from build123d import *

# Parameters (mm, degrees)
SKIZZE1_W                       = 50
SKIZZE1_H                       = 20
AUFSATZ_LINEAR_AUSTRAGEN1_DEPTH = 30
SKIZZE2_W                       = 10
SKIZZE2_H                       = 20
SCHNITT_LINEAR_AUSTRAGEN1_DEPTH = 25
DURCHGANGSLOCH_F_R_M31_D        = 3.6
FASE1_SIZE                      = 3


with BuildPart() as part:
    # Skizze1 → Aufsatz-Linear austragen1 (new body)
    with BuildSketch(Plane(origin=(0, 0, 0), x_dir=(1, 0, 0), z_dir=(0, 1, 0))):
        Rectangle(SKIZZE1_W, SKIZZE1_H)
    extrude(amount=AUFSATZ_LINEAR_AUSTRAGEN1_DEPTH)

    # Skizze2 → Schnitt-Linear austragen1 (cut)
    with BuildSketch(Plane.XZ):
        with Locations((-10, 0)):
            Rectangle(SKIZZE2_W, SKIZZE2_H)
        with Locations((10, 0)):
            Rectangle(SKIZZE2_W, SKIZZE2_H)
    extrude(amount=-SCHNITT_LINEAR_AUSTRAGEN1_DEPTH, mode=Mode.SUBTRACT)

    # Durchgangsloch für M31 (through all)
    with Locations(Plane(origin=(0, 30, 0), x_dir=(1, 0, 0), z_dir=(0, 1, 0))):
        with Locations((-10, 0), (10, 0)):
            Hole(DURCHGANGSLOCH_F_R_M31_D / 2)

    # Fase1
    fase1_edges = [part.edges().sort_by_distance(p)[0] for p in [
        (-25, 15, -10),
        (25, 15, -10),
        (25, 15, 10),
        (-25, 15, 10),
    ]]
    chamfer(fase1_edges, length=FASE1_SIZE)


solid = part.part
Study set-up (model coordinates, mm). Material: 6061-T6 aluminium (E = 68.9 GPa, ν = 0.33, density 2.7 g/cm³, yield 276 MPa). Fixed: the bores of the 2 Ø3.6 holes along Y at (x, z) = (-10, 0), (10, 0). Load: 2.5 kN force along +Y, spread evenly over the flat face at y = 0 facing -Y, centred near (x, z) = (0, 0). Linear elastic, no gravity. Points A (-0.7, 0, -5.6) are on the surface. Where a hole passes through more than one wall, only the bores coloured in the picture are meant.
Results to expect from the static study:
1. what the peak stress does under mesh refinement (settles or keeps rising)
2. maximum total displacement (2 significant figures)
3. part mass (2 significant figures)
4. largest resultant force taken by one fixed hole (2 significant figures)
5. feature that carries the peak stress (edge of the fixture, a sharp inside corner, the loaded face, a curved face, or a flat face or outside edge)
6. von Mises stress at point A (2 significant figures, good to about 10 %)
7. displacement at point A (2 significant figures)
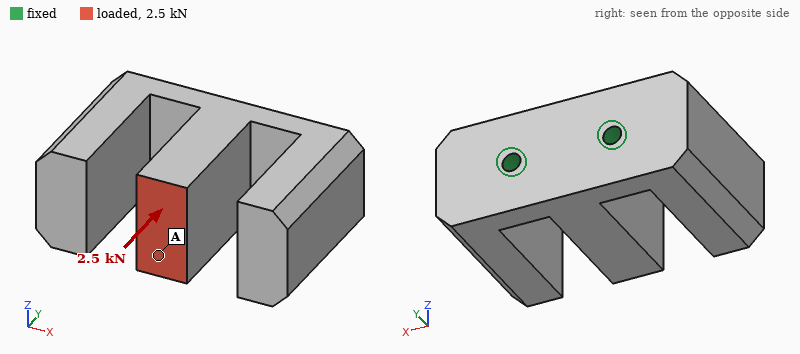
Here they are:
keeps rising
14 µm
52 g
1.3 kN
edge of the fixture
12 MPa
13 µm
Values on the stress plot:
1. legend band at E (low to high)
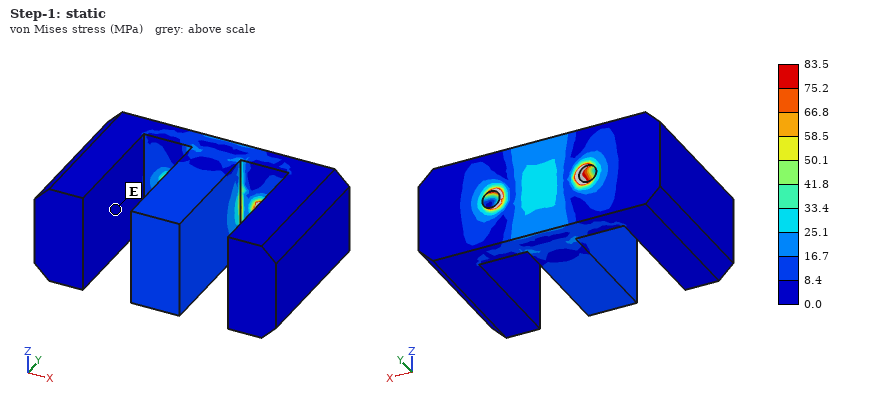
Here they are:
0.0 to 8.4 MPa
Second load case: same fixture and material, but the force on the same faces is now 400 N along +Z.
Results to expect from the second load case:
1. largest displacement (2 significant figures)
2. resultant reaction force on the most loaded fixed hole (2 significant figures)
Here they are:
56 µm
200 N
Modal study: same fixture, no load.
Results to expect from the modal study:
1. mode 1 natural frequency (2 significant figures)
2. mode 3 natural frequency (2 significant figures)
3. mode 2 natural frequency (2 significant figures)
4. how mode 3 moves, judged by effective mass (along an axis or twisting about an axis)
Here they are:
3200 Hz
4100 Hz
3200 Hz
along Z
